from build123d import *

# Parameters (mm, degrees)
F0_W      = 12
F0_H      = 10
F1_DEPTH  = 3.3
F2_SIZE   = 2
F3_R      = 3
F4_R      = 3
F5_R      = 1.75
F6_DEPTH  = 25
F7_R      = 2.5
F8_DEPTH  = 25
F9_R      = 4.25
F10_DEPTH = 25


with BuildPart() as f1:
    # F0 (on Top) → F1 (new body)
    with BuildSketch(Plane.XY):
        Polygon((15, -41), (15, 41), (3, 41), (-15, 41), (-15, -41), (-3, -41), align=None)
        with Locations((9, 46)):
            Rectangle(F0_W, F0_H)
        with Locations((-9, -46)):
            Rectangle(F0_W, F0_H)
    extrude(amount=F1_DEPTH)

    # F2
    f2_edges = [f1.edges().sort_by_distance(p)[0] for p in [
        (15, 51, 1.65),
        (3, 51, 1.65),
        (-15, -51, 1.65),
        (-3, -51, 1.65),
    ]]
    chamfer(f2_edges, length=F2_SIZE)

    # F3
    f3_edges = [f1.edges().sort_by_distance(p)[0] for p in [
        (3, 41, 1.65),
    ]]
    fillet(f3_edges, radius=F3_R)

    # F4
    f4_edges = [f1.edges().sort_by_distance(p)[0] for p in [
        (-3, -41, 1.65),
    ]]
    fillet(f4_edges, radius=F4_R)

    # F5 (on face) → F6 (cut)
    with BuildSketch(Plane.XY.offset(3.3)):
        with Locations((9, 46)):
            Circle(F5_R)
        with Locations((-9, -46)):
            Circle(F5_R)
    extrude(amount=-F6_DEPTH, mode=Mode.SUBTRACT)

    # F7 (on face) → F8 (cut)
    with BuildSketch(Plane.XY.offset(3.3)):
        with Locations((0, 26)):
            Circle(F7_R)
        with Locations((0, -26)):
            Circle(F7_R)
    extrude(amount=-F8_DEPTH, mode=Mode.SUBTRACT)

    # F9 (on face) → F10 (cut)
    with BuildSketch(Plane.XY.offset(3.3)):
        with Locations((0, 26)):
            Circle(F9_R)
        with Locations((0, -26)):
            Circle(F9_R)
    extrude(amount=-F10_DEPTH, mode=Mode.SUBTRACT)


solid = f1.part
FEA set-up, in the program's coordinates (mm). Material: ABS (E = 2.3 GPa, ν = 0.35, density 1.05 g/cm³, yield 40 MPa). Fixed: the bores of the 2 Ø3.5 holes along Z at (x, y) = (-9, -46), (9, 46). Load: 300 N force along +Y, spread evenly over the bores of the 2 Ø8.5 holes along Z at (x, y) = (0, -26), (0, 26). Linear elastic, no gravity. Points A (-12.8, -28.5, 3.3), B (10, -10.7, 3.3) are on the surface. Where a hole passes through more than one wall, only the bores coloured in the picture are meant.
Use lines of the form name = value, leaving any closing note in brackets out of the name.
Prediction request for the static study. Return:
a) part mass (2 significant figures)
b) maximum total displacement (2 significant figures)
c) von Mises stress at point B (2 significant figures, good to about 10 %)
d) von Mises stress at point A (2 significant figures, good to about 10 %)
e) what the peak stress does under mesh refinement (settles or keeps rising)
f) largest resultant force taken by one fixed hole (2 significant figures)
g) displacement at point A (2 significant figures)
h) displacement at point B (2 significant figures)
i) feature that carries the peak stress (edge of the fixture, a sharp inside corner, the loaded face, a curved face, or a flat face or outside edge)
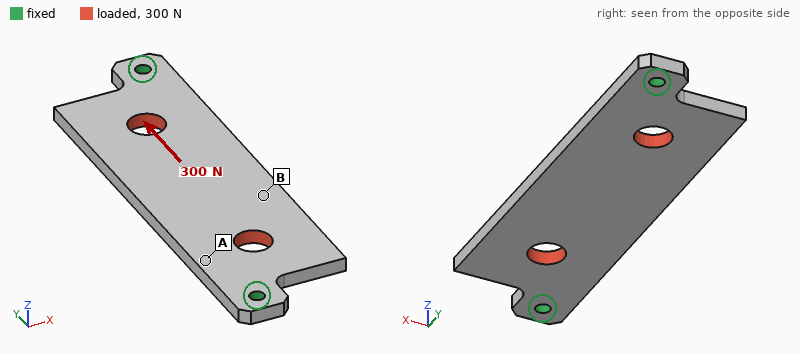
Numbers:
part mass = 8.9 g
maximum total displacement = 86 µm
von Mises stress at point B = 1.5 MPa
von Mises stress at point A = 2.9 MPa
what the peak stress does under mesh refinement = keeps rising
largest resultant force taken by one fixed hole = 150 N
displacement at point A = 42 µm
displacement at point B = 85 µm
feature that carries the peak stress = edge of the fixture
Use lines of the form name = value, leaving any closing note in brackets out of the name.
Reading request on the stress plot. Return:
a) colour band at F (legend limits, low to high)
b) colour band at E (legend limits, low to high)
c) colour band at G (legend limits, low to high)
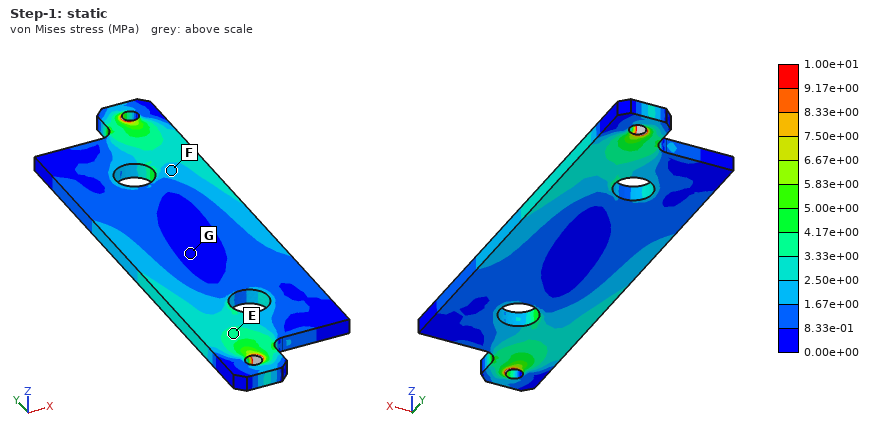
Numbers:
colour band at F = 1.67e+00 to 2.50e+00 MPa
colour band at E = 3.33e+00 to 4.17e+00 MPa
colour band at G = 0.00e+00 to 8.33e-01 MPa
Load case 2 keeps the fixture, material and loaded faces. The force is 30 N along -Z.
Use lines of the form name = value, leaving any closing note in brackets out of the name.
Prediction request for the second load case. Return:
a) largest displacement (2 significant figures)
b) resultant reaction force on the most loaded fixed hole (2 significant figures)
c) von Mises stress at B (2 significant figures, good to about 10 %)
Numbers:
largest displacement = 0.44 mm
resultant reaction force on the most loaded fixed hole = 15 N
von Mises stress at B = 1.9 MPa
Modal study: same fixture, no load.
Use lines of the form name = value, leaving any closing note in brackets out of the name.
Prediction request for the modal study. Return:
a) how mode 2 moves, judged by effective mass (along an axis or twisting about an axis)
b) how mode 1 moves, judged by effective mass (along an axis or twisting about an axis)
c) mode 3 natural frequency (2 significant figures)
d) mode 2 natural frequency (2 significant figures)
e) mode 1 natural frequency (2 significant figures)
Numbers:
how mode 2 moves, judged by effective mass = twisting about Y
how mode 1 moves, judged by effective mass = along Z
mode 3 natural frequency = 1400 Hz
mode 2 natural frequency = 690 Hz
mode 1 natural frequency = 470 Hz
